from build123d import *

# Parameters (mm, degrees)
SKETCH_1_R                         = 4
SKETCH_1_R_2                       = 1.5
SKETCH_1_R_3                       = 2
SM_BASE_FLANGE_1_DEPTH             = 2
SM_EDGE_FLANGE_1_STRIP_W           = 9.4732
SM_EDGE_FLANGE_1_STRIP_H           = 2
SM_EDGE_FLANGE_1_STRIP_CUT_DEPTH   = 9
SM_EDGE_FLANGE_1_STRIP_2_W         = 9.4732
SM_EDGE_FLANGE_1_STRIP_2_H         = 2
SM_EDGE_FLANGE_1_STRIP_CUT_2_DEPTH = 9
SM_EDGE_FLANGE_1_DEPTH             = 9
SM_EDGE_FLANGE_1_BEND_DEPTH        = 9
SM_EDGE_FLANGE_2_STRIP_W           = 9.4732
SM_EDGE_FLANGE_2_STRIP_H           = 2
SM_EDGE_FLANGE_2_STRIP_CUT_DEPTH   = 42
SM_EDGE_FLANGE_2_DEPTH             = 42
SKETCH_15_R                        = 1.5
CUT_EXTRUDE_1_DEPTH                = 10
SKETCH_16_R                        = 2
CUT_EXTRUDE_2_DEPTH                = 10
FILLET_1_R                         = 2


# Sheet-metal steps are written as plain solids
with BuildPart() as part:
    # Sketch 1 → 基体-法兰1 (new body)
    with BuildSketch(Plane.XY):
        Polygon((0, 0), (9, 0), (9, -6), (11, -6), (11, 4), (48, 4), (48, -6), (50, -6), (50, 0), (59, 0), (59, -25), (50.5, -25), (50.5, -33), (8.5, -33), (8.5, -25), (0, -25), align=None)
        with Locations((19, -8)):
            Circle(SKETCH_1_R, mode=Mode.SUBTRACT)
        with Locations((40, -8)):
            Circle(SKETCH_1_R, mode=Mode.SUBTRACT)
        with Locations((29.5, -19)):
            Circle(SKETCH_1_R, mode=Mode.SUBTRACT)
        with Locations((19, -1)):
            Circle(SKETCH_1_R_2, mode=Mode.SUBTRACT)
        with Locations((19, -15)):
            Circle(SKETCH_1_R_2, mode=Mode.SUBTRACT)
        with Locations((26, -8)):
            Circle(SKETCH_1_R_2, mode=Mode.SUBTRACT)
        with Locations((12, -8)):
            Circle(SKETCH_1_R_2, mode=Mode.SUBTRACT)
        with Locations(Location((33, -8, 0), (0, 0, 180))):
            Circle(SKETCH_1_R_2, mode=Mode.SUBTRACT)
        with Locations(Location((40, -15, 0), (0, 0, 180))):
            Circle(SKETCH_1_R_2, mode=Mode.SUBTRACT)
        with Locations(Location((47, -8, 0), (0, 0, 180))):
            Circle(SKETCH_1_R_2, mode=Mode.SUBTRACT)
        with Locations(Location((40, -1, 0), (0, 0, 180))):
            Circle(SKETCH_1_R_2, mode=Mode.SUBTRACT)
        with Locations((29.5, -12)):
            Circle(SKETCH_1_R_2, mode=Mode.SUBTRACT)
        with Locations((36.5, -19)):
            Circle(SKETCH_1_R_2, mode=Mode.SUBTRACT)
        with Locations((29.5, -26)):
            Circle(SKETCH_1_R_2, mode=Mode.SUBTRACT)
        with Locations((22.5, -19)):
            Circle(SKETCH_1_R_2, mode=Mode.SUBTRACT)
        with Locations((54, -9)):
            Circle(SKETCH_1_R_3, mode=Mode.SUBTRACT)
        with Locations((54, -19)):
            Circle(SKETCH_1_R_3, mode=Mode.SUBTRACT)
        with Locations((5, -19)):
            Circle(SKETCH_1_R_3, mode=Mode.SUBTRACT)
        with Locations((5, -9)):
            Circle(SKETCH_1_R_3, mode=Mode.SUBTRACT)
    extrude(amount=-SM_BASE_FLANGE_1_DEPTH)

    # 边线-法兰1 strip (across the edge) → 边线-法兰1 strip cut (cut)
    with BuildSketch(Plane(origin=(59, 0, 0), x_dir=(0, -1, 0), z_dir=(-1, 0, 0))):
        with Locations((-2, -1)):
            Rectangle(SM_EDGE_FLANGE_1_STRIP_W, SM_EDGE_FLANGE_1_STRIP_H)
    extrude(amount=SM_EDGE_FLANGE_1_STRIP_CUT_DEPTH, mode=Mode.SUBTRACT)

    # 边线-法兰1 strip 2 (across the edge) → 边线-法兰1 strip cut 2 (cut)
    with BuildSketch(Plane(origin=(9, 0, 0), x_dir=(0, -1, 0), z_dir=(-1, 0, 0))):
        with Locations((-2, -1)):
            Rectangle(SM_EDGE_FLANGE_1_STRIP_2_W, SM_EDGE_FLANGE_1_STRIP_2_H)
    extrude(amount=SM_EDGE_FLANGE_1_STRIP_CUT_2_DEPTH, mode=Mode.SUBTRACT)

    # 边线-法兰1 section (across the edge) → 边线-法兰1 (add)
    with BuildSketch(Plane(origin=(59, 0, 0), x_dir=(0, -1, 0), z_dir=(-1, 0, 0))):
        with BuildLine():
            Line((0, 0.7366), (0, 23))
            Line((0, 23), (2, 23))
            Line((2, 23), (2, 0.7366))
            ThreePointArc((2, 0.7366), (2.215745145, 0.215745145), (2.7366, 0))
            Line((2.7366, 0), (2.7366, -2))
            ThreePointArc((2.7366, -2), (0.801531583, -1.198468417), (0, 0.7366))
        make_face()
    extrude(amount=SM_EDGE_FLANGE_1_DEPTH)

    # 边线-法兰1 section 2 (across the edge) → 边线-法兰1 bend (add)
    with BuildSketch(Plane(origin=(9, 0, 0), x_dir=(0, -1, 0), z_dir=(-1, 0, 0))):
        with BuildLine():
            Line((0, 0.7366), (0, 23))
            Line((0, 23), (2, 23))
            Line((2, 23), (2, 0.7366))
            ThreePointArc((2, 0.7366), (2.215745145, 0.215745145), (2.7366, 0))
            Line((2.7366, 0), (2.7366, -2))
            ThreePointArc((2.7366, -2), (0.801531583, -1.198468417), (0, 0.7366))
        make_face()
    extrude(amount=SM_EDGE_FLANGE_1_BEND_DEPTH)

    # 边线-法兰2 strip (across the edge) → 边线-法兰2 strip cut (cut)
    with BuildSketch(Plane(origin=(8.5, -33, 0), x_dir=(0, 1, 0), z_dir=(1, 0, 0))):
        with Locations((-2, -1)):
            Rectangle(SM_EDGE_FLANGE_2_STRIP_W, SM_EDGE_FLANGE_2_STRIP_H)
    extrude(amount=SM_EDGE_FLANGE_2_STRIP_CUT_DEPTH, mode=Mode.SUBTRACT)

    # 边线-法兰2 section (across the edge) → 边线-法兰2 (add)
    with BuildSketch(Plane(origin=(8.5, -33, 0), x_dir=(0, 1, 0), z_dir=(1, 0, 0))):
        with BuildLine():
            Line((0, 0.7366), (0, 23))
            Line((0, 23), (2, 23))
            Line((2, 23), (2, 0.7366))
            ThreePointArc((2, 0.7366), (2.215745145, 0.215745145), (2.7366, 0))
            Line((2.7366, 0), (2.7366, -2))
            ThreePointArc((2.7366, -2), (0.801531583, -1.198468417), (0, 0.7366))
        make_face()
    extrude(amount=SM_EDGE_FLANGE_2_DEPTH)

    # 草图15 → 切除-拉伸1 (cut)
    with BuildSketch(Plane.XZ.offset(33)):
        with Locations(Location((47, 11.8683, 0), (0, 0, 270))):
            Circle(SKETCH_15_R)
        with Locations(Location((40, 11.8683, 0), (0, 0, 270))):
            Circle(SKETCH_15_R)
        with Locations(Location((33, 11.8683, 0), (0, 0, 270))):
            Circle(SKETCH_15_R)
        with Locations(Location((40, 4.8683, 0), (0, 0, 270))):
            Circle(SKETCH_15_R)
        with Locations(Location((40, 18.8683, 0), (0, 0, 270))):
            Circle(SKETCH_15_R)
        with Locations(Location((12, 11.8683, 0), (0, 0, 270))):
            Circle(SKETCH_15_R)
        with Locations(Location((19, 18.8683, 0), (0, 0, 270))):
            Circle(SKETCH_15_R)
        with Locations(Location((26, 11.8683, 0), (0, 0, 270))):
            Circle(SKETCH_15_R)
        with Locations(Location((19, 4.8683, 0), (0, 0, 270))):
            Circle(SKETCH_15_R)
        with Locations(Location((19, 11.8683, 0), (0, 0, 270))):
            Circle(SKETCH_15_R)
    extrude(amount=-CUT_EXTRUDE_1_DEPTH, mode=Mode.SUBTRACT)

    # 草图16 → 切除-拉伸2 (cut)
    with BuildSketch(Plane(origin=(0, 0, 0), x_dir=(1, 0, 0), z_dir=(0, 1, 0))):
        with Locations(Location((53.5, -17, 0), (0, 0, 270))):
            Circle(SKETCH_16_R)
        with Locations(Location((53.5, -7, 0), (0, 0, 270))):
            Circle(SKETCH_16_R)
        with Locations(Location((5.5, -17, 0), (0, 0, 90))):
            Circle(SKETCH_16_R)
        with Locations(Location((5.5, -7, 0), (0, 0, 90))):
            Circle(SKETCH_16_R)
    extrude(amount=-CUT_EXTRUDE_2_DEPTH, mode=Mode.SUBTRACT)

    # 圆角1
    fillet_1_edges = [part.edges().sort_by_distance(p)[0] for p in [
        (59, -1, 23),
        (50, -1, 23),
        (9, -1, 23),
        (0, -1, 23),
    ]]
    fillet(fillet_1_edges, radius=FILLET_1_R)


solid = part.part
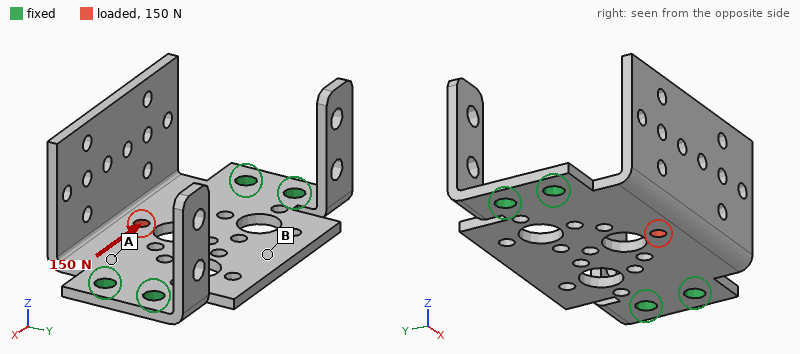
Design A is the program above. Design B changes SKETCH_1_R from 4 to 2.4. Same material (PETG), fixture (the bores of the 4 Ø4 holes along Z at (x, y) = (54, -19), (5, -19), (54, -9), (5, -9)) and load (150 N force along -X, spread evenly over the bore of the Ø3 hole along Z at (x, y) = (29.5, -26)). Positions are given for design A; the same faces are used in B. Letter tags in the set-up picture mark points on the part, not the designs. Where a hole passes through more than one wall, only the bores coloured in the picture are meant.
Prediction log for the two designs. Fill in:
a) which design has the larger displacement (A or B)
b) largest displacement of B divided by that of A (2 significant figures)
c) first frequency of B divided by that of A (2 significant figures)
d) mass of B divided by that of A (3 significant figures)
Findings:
A
0.91
1.0
1.03
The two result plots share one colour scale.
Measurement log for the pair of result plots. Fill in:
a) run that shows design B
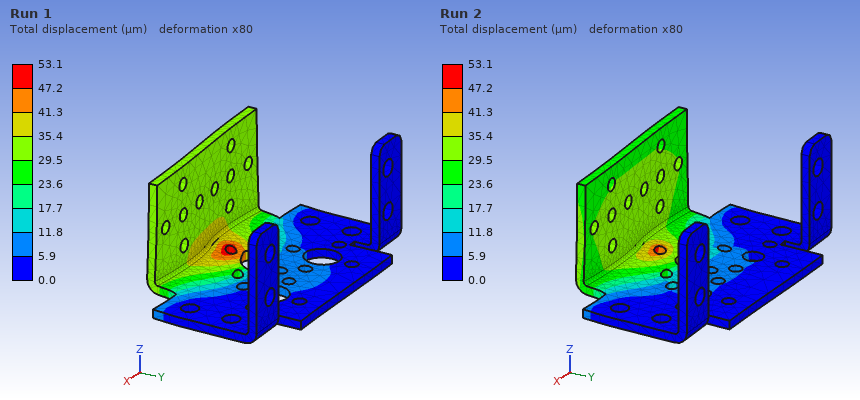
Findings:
Run 2
